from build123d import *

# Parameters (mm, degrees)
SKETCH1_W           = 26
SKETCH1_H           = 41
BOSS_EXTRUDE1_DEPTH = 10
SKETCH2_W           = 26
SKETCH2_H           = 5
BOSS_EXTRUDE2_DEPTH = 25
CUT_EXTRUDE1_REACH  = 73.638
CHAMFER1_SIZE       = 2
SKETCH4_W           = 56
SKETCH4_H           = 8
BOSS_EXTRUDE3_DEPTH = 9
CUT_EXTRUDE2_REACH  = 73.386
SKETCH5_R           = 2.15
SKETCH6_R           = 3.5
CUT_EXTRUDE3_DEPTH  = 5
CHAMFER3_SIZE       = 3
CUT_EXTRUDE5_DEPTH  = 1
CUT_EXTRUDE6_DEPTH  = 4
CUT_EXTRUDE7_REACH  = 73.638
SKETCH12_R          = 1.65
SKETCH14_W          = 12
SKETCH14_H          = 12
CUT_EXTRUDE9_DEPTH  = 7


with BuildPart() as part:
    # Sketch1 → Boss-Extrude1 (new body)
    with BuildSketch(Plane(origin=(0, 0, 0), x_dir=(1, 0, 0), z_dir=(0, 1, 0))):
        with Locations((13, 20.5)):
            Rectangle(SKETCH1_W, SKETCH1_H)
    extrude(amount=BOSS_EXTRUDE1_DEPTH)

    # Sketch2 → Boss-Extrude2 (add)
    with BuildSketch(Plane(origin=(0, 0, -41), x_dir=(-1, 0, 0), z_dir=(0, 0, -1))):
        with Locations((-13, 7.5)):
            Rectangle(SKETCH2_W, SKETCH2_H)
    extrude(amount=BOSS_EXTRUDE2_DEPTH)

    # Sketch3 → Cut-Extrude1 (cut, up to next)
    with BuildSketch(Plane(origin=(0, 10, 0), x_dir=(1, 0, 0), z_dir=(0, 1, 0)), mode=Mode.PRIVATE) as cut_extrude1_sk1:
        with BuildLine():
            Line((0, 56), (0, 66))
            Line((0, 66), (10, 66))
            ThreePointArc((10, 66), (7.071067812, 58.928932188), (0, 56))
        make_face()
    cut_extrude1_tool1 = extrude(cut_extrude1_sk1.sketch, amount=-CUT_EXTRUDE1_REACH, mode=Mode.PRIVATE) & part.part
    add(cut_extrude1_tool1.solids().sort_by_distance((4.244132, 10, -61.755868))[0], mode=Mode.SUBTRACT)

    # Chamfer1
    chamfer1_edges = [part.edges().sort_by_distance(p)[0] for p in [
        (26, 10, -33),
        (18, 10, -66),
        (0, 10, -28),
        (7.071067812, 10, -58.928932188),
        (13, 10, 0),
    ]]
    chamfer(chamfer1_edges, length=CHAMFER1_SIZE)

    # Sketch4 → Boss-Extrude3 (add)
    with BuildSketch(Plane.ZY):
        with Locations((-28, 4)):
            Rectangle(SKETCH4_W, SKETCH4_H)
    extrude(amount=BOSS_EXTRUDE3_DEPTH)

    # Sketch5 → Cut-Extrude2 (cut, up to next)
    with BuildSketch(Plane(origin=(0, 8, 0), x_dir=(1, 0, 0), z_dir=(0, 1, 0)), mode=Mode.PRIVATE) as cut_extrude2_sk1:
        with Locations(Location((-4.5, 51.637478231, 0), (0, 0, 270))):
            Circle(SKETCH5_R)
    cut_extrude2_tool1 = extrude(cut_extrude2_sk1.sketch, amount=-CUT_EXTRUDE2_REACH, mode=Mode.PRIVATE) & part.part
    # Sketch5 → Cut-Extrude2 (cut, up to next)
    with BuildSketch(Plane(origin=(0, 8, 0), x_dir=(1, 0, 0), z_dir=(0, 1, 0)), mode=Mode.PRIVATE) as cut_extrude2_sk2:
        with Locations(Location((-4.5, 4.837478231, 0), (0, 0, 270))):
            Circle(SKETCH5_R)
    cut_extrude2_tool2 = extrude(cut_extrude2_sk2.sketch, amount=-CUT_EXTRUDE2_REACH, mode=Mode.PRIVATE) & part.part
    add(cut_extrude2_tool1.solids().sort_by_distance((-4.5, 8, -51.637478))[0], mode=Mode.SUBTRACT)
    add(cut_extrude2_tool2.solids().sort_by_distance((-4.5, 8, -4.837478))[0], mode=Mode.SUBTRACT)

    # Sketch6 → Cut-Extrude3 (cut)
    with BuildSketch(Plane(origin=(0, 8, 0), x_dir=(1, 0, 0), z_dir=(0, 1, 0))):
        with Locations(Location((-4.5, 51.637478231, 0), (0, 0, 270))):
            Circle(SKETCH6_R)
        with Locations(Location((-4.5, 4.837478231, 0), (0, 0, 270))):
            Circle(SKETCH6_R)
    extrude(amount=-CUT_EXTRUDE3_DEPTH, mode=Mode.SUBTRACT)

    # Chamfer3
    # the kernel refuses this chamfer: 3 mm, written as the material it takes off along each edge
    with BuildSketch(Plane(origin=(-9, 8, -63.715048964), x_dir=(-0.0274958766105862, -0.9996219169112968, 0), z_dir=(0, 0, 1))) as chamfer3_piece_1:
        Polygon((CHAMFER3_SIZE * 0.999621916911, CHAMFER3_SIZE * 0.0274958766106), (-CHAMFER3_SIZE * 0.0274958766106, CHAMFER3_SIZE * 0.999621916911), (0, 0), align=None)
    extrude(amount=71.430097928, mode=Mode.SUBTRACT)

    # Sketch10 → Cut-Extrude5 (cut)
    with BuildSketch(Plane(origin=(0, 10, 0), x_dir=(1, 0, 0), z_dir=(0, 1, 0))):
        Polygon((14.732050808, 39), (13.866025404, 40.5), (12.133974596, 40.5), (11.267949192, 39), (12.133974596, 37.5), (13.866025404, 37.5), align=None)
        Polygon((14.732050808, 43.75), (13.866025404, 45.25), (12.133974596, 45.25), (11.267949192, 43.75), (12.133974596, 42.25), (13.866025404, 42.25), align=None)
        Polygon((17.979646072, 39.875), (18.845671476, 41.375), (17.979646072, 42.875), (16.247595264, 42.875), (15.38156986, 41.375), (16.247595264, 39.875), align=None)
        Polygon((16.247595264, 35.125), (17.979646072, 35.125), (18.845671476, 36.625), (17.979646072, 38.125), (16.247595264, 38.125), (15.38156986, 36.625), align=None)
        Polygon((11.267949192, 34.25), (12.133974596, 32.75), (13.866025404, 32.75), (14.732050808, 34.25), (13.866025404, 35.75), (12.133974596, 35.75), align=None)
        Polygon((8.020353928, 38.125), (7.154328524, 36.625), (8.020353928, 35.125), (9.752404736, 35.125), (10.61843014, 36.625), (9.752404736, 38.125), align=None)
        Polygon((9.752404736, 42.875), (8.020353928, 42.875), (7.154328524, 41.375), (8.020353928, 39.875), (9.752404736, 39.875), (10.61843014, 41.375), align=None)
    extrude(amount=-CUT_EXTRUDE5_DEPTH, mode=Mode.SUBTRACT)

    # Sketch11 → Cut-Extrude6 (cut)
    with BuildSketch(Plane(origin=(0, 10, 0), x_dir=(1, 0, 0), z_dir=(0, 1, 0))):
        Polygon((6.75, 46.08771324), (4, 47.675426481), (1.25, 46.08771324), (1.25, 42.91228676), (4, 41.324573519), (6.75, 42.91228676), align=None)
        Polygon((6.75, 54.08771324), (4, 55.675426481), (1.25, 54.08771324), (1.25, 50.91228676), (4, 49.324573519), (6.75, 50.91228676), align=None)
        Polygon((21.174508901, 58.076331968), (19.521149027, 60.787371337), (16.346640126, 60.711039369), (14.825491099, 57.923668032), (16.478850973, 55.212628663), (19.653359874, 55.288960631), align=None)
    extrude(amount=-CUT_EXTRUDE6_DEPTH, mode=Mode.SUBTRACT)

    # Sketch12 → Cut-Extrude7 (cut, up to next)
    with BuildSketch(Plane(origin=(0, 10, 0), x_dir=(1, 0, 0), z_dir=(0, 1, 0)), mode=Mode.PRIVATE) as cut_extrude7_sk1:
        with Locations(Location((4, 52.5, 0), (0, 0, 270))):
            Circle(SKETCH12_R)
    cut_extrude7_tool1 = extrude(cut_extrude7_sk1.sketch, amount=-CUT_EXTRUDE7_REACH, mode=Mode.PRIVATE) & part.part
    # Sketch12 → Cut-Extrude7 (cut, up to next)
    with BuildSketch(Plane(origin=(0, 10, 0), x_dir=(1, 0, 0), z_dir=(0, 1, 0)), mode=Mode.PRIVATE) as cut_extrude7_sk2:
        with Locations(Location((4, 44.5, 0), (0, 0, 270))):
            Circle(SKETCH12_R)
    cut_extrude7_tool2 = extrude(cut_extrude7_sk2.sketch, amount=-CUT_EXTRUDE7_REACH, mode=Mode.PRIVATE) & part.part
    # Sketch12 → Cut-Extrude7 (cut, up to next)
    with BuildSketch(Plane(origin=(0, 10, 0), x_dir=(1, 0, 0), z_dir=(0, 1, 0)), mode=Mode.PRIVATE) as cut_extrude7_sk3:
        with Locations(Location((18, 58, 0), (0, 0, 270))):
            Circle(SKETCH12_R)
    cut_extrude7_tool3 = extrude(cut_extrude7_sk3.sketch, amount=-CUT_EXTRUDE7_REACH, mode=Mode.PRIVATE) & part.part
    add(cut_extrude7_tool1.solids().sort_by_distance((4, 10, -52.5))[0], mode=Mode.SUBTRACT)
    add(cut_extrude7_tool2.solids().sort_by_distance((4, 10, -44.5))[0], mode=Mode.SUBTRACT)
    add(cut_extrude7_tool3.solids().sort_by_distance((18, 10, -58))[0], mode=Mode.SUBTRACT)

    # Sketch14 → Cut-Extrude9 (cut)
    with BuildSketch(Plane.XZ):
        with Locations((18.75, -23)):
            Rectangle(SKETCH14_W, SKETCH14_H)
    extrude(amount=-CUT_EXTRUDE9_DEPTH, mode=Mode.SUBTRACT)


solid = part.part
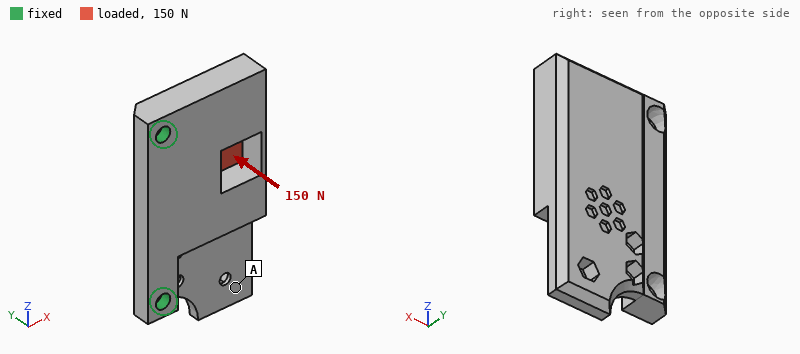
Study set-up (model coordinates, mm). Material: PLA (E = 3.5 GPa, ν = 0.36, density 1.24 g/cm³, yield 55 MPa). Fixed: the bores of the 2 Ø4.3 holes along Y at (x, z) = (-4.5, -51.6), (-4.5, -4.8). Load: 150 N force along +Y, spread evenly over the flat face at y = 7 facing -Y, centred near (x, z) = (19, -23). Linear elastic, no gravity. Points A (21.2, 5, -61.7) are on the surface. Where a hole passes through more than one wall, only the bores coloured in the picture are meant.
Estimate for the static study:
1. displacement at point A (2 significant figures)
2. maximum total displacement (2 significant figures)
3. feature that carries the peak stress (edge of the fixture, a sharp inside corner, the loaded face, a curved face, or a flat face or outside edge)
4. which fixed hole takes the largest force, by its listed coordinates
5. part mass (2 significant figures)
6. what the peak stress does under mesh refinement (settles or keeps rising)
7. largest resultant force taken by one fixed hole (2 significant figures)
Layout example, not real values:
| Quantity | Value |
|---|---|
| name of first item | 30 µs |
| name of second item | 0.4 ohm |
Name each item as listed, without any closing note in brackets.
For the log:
| Quantity | Value |
|---|---|
| displacement at point A | 0.60 mm |
| maximum total displacement | 0.84 mm |
| feature that carries the peak stress | edge of the fixture |
| which fixed hole takes the largest force, by its listed coordinates | (-4.5, -4.8) |
| part mass | 19 g |
| what the peak stress does under mesh refinement | keeps rising |
| largest resultant force taken by one fixed hole | 110 N |
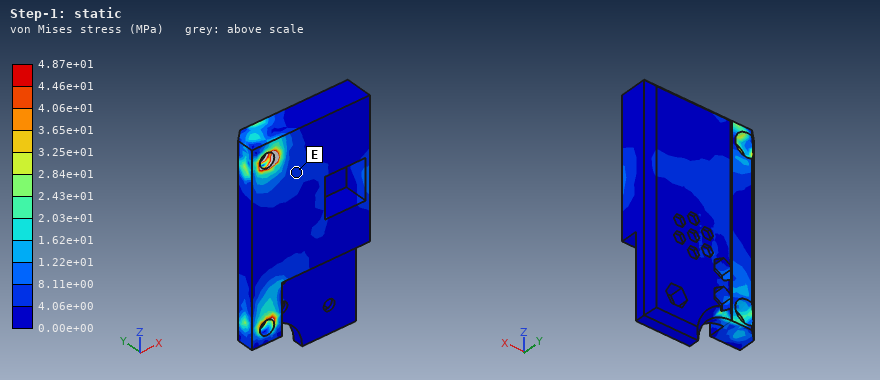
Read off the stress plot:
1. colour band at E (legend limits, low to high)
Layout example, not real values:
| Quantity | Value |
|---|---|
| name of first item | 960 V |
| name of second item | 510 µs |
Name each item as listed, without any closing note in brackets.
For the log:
| Quantity | Value |
|---|---|
| colour band at E | 4.06e+00 to 8.11e+00 MPa |
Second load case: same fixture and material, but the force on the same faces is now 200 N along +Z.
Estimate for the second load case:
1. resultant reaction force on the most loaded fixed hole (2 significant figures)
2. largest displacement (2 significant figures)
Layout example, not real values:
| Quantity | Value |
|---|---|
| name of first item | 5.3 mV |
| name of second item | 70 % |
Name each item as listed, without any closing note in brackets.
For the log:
| Quantity | Value |
|---|---|
| resultant reaction force on the most loaded fixed hole | 150 N |
| largest displacement | 59 µm |
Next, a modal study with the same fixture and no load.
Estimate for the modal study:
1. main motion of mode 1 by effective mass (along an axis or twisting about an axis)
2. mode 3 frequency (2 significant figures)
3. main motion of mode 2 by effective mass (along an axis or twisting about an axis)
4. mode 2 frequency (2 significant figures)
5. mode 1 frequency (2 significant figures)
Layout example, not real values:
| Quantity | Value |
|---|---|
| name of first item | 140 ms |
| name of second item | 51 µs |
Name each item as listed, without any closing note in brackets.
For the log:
| Quantity | Value |
|---|---|
| main motion of mode 1 by effective mass | along Y |
| mode 3 frequency | 3200 Hz |
| main motion of mode 2 by effective mass | twisting about X |
| mode 2 frequency | 1900 Hz |
| mode 1 frequency | 800 Hz |
